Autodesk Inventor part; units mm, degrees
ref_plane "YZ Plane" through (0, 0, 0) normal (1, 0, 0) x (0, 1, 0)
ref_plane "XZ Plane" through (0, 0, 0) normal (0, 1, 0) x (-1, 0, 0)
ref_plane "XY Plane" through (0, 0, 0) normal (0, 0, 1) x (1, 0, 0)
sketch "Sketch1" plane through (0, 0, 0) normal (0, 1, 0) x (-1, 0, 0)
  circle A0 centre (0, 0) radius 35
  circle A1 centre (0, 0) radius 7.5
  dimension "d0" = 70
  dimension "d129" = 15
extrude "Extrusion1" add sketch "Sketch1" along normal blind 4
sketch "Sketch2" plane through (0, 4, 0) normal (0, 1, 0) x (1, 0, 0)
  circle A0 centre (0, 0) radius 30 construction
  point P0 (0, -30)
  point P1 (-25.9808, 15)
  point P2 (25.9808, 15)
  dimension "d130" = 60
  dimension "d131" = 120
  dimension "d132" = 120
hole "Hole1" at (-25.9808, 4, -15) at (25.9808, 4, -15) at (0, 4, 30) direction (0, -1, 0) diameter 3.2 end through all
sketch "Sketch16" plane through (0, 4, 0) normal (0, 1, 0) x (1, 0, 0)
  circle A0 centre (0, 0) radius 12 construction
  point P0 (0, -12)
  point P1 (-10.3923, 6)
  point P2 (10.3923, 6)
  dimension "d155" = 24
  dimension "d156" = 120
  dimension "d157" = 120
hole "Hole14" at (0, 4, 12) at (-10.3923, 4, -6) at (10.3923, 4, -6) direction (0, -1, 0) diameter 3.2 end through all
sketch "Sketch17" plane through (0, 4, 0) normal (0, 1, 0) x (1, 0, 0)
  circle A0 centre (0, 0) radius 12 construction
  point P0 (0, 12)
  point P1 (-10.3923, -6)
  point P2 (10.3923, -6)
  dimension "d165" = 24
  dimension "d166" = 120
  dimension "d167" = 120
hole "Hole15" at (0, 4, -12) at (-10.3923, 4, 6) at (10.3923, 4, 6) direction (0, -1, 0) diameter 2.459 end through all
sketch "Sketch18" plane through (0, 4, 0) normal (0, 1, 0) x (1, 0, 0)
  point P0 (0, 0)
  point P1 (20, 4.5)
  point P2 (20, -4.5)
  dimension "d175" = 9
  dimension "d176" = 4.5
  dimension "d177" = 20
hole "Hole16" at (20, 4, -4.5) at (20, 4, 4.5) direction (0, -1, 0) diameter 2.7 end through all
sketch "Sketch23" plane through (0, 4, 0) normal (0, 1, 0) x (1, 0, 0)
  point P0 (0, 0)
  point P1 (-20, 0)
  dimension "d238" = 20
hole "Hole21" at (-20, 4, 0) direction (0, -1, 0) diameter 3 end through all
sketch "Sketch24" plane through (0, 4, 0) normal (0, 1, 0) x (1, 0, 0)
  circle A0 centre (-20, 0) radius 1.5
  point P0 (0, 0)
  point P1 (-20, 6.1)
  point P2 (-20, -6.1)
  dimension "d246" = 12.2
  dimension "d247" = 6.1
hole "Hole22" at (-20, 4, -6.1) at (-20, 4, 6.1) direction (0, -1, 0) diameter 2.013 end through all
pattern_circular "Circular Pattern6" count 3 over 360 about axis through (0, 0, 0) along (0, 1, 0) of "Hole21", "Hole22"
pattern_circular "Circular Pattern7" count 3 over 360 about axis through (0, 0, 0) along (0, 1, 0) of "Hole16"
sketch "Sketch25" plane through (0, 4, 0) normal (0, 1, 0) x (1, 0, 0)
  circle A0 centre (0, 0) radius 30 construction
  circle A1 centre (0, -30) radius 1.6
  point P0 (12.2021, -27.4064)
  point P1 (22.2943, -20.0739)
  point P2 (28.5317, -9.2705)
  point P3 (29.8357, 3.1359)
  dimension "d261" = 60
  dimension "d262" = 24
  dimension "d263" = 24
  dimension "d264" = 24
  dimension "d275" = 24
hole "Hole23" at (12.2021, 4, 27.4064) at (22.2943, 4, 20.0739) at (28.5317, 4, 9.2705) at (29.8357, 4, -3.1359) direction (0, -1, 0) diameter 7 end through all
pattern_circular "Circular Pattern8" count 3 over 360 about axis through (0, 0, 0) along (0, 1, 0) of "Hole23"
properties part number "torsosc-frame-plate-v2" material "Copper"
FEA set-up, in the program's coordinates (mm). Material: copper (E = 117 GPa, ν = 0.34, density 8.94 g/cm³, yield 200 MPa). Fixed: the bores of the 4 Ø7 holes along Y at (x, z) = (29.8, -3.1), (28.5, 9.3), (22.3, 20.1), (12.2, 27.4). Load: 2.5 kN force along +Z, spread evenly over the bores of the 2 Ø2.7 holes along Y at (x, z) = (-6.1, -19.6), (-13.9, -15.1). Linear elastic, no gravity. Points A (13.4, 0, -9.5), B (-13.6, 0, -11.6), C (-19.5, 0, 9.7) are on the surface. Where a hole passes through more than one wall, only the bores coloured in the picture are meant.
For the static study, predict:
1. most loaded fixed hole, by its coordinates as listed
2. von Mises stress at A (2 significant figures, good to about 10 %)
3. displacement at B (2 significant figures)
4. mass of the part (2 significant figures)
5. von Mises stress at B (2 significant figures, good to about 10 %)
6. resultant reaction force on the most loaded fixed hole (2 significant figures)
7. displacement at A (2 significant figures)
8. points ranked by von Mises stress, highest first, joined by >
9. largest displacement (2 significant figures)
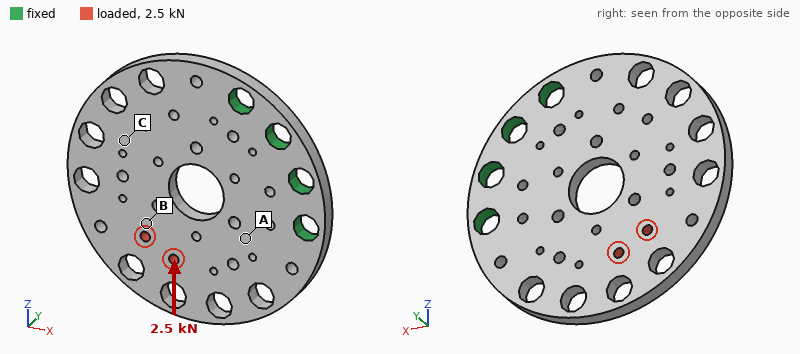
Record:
(12.2, 27.4)
28 MPa
29 µm
110 g
50 MPa
2.4 kN
8.6 µm
B > A > C
34 µm
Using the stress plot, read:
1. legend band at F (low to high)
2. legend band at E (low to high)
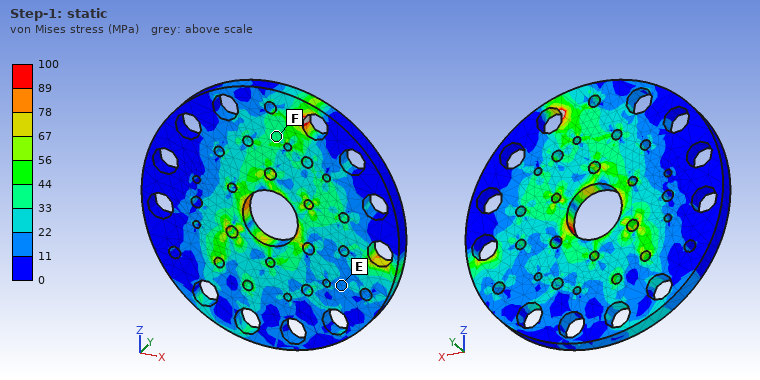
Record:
33 to 44 MPa
11 to 22 MPa
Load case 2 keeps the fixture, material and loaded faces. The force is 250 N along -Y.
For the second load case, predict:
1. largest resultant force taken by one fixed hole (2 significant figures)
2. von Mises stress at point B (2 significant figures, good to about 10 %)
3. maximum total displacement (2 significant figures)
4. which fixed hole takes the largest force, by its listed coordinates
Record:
250 N
21 MPa
0.32 mm
(29.8, -3.1)
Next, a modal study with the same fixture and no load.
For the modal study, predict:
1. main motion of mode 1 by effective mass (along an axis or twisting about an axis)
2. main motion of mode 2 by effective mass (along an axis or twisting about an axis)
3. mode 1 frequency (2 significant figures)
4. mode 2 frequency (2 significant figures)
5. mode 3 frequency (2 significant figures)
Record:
along Y
twisting about X
810 Hz
1900 Hz
3800 Hz
